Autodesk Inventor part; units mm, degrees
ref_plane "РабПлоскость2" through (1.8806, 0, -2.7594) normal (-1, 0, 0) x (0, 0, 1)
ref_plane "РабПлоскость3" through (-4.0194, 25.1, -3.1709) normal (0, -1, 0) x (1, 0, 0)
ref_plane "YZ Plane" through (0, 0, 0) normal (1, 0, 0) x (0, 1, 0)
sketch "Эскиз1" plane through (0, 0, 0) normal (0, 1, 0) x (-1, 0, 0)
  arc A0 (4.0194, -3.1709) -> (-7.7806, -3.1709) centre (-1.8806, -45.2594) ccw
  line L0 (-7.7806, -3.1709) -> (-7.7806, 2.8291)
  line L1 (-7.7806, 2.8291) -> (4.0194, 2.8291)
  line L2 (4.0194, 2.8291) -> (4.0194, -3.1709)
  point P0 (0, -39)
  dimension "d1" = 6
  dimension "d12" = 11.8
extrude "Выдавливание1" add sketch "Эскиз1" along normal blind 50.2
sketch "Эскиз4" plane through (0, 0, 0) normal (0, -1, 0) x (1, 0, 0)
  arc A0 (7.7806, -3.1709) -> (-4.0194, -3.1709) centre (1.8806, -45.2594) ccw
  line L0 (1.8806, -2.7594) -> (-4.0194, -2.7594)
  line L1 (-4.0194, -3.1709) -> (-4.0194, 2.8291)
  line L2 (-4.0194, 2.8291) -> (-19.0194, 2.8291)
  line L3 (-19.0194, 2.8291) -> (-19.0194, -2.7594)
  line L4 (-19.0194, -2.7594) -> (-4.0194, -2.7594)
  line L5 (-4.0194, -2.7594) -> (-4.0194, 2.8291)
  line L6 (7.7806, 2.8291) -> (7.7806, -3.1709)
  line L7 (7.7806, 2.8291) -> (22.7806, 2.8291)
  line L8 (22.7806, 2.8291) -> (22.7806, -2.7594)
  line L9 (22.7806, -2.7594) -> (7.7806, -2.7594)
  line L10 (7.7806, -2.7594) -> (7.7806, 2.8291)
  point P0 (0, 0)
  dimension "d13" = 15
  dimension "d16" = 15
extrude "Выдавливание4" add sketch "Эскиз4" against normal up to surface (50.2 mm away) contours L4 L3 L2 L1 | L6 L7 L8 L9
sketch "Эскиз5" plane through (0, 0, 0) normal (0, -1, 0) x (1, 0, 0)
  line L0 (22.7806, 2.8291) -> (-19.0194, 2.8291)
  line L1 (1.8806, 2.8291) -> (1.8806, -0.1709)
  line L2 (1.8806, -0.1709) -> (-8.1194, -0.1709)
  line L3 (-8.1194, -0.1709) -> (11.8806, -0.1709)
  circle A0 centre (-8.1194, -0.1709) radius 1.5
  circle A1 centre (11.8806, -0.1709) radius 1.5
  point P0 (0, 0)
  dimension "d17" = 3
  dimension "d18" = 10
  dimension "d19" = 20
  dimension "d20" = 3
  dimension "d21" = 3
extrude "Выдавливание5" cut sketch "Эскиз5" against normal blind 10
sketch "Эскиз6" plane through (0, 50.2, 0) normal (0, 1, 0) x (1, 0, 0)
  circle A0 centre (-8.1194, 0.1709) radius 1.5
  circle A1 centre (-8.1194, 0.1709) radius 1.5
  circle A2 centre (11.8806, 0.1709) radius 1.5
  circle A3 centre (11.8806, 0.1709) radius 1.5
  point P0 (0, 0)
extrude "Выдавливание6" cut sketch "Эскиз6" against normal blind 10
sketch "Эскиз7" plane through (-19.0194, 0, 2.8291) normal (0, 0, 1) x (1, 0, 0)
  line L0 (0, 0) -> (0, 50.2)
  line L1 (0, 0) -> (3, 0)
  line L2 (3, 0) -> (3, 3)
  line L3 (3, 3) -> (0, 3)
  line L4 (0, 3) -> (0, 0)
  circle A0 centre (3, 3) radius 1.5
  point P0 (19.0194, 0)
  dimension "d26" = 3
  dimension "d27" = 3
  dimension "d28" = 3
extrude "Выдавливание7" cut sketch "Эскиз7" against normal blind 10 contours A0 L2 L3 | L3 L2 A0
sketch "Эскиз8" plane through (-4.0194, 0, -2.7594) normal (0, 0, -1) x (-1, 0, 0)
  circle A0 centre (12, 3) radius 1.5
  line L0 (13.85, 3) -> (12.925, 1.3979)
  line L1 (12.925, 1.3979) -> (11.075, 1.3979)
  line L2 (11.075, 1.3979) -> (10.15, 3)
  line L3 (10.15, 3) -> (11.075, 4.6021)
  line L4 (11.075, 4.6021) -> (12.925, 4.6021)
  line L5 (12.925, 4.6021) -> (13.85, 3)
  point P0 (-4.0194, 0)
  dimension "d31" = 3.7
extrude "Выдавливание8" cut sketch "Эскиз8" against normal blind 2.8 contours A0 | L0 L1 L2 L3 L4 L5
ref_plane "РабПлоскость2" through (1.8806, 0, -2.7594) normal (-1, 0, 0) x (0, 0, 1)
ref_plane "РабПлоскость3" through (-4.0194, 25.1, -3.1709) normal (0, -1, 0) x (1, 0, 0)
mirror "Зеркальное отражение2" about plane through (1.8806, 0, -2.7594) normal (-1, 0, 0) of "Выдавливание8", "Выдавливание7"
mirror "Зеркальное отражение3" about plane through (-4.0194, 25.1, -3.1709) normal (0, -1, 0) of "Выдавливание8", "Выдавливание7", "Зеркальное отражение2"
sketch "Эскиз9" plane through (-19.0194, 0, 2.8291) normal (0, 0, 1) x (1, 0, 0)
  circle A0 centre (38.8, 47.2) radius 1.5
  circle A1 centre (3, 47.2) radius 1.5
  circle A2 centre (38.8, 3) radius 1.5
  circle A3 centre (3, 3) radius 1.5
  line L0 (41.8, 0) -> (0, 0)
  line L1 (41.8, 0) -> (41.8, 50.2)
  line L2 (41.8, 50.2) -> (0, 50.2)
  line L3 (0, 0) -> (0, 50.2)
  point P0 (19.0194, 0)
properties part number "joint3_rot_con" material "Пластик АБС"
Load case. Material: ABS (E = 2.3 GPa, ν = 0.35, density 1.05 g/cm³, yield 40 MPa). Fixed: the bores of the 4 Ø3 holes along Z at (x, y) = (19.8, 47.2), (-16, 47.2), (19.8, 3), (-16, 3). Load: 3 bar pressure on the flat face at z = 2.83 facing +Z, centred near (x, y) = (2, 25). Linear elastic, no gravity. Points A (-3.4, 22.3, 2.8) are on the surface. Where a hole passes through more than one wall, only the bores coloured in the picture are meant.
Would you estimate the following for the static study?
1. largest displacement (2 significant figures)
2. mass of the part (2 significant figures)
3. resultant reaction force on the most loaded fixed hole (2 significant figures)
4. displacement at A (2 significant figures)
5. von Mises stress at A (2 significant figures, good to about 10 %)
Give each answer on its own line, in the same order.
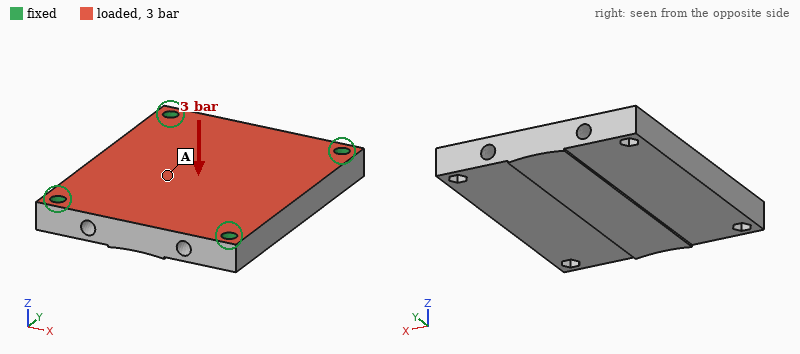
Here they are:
0.27 mm
12 g
190 N
0.26 mm
5.6 MPa
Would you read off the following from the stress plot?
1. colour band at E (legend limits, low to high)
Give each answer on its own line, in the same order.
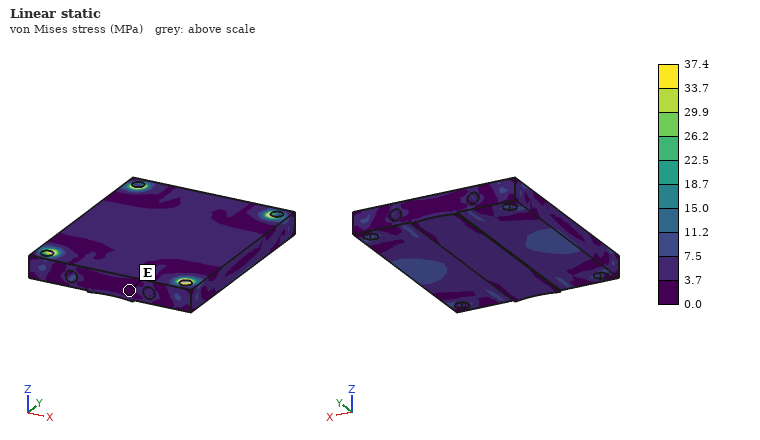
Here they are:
0.0 to 3.7 MPa
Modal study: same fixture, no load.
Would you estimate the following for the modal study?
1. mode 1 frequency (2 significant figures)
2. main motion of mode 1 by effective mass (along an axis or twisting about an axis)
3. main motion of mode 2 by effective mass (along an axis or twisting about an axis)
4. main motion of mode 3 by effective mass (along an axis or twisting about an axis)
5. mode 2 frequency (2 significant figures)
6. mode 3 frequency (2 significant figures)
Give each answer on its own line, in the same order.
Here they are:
2500 Hz
along Z
twisting about Y
twisting about X
4000 Hz
4800 Hz
